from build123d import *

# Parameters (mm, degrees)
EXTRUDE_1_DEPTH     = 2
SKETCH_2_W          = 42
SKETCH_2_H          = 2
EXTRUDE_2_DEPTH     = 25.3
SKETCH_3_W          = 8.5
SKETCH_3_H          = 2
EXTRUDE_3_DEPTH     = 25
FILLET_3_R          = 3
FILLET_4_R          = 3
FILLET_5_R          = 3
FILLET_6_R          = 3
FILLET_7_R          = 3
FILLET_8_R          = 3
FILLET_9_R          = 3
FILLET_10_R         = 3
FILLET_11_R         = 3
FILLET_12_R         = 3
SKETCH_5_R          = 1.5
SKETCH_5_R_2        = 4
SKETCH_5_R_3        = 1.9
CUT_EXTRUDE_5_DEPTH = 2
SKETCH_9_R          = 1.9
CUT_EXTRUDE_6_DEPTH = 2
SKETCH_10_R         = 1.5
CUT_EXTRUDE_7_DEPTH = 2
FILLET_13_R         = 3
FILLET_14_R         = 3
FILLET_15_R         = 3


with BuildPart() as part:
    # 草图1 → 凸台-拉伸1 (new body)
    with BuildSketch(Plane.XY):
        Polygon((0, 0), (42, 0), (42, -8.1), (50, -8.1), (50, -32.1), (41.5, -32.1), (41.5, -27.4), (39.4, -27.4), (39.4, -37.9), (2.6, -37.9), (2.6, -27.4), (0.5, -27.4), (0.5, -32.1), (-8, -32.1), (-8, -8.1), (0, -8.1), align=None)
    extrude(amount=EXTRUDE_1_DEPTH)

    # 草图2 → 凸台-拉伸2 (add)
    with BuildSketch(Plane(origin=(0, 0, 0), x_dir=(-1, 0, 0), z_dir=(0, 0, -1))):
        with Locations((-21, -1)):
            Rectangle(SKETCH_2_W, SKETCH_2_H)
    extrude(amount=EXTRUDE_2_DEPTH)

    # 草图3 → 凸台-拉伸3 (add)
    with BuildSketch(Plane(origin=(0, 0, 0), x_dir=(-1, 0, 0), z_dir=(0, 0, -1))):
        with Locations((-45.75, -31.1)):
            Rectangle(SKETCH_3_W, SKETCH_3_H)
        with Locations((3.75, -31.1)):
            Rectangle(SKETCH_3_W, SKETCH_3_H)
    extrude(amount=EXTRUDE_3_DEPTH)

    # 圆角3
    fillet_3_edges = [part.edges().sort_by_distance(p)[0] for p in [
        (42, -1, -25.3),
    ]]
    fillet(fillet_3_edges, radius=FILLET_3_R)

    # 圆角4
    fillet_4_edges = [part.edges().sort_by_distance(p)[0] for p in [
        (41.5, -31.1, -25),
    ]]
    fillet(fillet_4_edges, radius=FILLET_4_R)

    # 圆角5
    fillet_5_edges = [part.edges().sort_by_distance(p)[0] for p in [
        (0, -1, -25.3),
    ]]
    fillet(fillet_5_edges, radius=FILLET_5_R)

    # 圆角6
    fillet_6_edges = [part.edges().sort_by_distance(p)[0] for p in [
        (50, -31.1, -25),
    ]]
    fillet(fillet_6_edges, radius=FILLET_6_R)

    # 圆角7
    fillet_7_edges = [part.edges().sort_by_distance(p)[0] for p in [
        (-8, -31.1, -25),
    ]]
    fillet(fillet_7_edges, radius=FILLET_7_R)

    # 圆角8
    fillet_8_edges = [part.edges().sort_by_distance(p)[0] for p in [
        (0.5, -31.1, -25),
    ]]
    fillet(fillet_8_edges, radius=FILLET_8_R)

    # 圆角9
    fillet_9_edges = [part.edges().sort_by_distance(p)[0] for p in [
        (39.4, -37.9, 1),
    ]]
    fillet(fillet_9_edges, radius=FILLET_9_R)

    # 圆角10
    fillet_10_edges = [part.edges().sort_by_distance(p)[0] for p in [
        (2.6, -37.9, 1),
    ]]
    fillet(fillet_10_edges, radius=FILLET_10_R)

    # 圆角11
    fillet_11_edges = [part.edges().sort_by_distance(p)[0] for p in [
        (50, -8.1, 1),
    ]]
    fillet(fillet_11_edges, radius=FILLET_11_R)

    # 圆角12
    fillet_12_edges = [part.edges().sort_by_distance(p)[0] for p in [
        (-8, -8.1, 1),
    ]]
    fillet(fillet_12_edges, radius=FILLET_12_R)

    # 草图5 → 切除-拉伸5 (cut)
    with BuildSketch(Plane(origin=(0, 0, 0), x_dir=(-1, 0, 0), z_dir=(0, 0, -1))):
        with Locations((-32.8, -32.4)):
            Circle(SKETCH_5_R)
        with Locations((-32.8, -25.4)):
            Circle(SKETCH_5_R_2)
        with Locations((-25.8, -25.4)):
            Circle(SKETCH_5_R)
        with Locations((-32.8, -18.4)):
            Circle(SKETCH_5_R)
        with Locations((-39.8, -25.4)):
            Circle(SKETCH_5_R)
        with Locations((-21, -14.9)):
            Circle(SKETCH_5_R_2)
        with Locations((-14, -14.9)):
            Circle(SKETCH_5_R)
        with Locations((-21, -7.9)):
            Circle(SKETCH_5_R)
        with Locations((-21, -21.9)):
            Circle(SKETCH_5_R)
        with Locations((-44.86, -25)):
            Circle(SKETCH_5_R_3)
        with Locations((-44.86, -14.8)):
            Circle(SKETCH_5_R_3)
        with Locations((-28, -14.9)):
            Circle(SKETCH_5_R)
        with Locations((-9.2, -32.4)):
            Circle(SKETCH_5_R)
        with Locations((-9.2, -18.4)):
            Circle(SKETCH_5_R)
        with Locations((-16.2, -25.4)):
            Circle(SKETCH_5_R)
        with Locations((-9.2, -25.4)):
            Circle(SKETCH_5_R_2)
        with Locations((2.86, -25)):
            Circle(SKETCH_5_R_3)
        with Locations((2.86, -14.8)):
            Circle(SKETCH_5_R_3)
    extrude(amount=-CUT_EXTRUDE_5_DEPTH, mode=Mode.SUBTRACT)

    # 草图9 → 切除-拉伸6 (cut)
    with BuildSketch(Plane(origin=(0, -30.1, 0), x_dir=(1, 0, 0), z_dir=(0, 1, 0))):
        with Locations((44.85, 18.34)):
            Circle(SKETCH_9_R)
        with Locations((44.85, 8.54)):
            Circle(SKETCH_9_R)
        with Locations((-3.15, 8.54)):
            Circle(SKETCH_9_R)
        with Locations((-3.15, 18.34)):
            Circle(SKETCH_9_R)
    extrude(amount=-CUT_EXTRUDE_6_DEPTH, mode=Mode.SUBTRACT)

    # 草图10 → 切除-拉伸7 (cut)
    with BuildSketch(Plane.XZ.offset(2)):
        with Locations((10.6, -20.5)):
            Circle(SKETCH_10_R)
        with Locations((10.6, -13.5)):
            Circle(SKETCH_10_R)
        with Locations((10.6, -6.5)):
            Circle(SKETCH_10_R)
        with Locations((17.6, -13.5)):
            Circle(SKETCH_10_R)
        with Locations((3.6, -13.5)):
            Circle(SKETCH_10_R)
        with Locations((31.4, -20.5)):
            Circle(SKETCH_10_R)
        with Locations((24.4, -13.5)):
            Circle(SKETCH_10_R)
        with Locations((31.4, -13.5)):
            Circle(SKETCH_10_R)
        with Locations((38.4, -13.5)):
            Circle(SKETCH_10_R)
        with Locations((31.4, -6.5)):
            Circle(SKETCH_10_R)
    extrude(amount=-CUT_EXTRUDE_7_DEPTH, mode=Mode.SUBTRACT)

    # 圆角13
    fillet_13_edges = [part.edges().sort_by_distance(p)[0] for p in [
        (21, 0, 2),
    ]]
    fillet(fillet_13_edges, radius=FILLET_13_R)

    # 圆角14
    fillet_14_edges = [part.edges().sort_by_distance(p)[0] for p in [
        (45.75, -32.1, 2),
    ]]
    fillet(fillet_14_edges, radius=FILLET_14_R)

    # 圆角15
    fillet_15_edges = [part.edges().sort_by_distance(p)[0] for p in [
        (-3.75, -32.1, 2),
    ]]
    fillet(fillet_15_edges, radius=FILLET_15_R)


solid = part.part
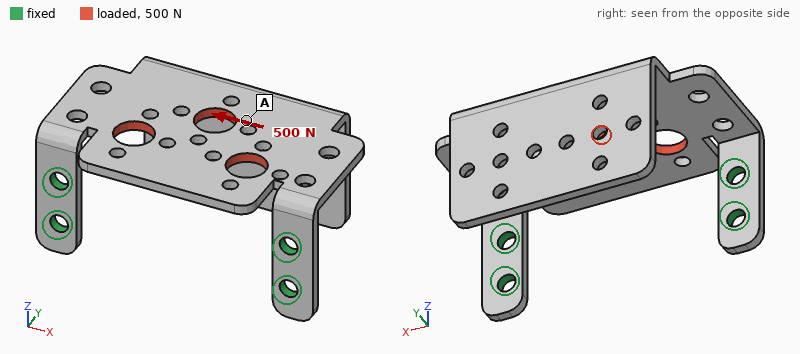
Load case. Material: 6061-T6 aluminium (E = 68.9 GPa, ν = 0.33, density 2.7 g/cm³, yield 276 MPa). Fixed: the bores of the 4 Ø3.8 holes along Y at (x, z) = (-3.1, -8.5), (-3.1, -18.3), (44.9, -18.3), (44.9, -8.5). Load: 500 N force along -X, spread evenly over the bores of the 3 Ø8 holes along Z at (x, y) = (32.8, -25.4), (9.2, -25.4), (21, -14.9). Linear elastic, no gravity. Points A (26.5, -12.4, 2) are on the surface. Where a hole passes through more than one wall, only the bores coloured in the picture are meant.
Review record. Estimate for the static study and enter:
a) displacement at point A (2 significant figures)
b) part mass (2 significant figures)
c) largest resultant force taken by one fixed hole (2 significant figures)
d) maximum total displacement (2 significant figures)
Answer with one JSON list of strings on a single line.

["0.057 mm", "16 g", "340 N", "0.14 mm"]
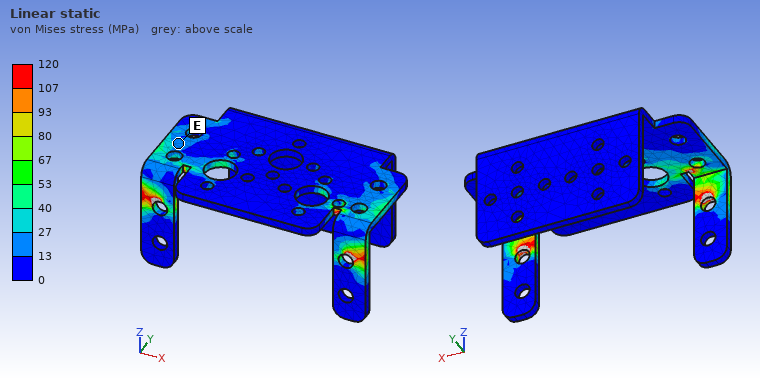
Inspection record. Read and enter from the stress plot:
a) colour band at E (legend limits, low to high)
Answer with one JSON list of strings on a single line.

["13 to 27 MPa"]
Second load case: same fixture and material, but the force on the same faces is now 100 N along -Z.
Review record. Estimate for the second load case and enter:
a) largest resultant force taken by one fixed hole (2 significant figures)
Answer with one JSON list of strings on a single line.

["52 N"]
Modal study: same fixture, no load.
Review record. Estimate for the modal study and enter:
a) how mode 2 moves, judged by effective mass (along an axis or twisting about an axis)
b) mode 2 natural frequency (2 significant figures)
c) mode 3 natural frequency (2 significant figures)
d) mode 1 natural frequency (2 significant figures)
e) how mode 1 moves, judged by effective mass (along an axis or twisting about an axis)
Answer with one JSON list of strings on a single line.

["along X", "1100 Hz", "1400 Hz", "360 Hz", "along Z"]
